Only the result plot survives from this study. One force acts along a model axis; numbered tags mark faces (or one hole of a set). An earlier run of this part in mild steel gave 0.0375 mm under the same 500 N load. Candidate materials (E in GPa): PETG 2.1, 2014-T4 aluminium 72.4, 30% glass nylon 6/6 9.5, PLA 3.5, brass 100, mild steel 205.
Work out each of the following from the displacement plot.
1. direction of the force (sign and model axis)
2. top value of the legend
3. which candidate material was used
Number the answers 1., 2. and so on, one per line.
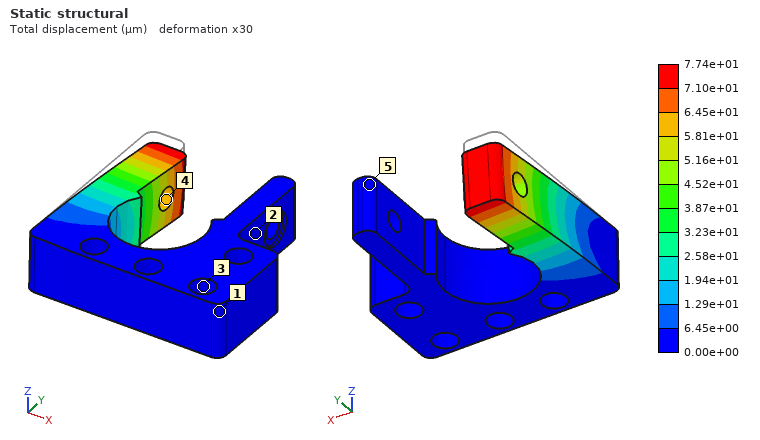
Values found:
1. -Z
2. 7.74e+01 µm
3. brass
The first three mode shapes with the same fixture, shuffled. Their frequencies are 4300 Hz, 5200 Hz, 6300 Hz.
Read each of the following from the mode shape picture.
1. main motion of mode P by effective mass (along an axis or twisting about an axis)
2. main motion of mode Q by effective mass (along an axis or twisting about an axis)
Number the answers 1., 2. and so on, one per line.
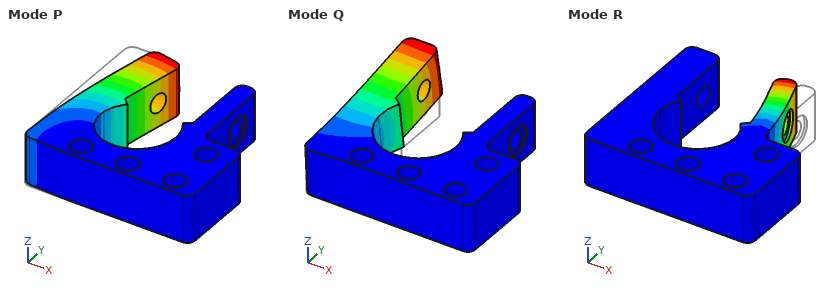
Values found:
1. along X
2. along Z
